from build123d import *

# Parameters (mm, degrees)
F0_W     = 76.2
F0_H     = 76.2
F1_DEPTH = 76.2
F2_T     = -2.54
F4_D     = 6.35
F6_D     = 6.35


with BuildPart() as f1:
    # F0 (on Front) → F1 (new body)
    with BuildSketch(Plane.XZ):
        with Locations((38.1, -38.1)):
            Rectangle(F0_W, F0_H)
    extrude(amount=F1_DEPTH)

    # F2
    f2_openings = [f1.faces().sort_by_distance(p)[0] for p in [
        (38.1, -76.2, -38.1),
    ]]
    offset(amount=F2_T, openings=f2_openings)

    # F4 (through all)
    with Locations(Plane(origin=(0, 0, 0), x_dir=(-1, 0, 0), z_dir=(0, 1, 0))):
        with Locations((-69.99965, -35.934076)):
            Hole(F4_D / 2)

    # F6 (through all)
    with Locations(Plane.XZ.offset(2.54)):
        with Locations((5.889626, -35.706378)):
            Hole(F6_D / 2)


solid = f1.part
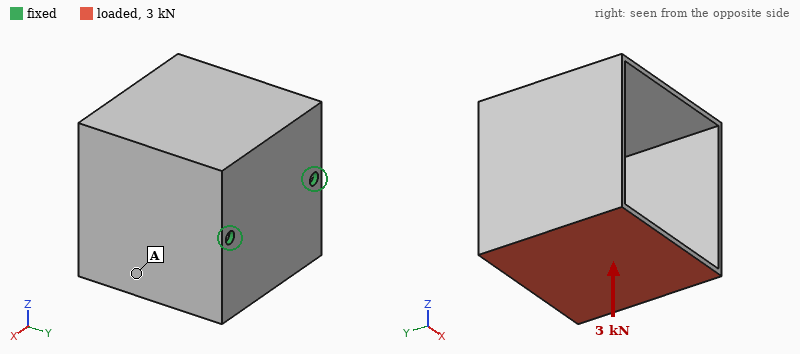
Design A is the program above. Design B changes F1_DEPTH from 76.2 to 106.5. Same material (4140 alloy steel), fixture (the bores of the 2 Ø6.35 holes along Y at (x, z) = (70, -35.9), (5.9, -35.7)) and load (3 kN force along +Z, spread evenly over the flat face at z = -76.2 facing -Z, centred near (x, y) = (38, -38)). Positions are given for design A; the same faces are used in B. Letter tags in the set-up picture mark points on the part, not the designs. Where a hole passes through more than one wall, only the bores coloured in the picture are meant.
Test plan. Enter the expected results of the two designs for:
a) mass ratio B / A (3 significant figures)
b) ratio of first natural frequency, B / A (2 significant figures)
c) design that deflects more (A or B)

1.33
0.67
B
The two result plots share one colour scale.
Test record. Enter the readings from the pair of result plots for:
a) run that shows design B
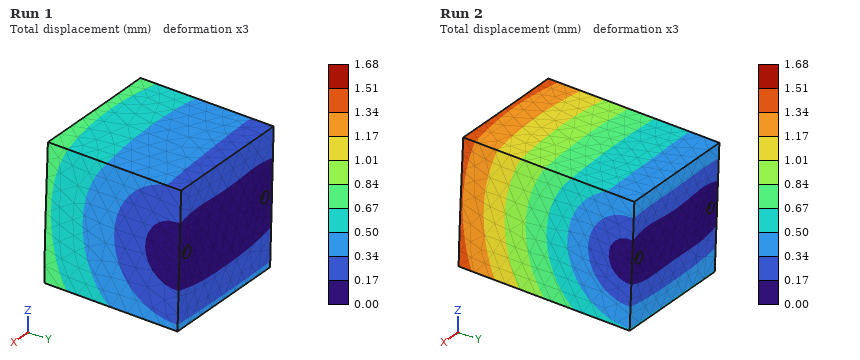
Run 2
